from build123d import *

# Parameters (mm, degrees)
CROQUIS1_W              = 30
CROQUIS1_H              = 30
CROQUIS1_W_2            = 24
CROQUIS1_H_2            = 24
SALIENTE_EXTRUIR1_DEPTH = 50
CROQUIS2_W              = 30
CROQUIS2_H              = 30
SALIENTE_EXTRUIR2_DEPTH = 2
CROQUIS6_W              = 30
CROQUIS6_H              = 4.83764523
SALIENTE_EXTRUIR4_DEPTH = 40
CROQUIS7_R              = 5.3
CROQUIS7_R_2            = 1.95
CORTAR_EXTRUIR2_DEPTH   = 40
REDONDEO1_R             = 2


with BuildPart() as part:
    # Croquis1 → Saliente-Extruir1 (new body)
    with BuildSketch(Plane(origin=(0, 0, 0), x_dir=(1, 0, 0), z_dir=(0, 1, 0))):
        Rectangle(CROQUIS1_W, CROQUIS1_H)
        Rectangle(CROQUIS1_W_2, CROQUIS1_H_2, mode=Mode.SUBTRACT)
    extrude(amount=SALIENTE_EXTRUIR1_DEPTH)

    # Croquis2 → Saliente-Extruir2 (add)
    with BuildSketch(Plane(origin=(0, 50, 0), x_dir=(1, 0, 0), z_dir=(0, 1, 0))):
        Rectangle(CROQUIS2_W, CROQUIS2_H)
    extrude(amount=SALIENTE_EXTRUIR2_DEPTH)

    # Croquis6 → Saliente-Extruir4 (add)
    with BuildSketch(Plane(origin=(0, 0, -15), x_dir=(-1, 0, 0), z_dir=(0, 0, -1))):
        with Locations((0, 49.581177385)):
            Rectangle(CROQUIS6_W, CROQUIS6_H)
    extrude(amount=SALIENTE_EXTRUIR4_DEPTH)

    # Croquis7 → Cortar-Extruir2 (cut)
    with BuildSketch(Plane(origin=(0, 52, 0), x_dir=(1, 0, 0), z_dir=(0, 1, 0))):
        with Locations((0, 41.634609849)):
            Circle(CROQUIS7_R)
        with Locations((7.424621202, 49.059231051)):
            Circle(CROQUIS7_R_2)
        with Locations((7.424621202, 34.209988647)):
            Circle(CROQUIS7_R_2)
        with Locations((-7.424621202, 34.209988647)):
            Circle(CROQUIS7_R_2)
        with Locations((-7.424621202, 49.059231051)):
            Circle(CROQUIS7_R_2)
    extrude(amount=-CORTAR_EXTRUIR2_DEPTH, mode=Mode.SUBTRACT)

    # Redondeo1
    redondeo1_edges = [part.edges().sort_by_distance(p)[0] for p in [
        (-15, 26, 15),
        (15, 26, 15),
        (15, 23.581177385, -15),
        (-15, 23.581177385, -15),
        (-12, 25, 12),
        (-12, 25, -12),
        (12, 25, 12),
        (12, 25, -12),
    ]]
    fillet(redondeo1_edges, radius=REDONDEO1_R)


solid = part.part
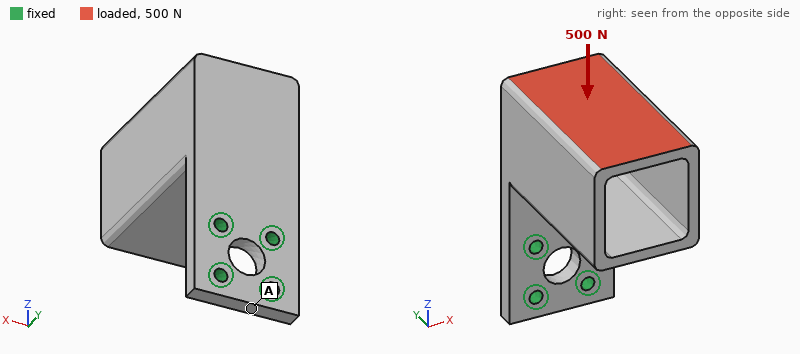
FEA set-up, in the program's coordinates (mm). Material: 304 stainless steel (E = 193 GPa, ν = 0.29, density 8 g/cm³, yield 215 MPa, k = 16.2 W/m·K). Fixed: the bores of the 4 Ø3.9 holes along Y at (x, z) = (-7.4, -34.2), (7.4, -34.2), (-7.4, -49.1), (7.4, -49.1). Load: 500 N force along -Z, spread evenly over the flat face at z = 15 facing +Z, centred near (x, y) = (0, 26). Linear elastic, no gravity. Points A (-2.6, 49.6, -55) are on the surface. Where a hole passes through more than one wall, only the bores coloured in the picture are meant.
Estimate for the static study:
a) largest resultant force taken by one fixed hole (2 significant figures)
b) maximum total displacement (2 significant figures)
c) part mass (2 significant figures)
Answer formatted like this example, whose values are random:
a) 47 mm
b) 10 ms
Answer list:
a) 230 N
b) 0.33 mm
c) 190 g
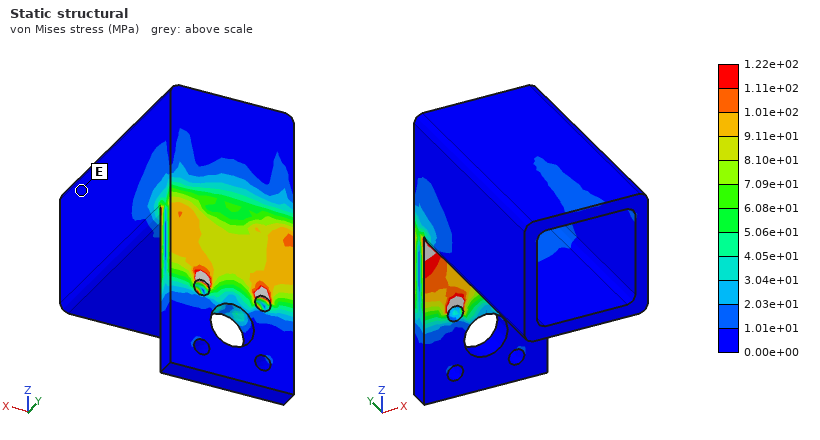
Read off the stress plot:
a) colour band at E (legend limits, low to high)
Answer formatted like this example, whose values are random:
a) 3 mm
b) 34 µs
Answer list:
a) 0.00e+00 to 1.01e+01 MPa
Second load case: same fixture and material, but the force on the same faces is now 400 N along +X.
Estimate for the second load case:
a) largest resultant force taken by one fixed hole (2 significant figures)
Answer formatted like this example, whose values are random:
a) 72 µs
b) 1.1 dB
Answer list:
a) 1.0 kN
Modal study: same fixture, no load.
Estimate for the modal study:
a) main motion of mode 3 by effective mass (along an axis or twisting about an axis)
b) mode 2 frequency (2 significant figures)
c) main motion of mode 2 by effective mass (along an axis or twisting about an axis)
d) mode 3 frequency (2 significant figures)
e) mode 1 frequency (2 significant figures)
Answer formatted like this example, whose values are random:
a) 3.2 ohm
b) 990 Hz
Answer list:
a) along Y
b) 1100 Hz
c) along X
d) 3400 Hz
e) 540 Hz
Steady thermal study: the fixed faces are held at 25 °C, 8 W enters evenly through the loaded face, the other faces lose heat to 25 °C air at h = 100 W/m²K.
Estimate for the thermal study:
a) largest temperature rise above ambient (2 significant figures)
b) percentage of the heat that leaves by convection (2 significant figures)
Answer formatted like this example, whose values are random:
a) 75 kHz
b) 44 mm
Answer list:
a) 21 K
b) 98 %
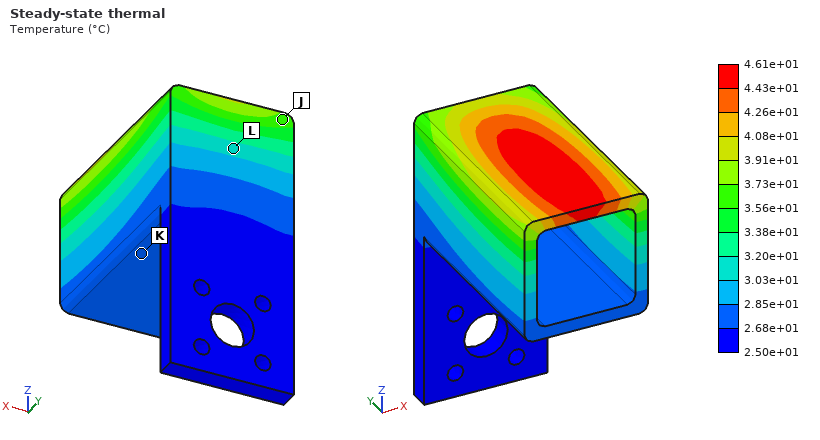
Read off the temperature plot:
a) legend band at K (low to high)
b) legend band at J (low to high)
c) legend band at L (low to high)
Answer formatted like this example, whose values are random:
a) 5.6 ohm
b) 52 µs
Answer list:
a) 2.68e+01 to 2.85e+01 °C
b) 3.56e+01 to 3.73e+01 °C
c) 3.03e+01 to 3.20e+01 °C
